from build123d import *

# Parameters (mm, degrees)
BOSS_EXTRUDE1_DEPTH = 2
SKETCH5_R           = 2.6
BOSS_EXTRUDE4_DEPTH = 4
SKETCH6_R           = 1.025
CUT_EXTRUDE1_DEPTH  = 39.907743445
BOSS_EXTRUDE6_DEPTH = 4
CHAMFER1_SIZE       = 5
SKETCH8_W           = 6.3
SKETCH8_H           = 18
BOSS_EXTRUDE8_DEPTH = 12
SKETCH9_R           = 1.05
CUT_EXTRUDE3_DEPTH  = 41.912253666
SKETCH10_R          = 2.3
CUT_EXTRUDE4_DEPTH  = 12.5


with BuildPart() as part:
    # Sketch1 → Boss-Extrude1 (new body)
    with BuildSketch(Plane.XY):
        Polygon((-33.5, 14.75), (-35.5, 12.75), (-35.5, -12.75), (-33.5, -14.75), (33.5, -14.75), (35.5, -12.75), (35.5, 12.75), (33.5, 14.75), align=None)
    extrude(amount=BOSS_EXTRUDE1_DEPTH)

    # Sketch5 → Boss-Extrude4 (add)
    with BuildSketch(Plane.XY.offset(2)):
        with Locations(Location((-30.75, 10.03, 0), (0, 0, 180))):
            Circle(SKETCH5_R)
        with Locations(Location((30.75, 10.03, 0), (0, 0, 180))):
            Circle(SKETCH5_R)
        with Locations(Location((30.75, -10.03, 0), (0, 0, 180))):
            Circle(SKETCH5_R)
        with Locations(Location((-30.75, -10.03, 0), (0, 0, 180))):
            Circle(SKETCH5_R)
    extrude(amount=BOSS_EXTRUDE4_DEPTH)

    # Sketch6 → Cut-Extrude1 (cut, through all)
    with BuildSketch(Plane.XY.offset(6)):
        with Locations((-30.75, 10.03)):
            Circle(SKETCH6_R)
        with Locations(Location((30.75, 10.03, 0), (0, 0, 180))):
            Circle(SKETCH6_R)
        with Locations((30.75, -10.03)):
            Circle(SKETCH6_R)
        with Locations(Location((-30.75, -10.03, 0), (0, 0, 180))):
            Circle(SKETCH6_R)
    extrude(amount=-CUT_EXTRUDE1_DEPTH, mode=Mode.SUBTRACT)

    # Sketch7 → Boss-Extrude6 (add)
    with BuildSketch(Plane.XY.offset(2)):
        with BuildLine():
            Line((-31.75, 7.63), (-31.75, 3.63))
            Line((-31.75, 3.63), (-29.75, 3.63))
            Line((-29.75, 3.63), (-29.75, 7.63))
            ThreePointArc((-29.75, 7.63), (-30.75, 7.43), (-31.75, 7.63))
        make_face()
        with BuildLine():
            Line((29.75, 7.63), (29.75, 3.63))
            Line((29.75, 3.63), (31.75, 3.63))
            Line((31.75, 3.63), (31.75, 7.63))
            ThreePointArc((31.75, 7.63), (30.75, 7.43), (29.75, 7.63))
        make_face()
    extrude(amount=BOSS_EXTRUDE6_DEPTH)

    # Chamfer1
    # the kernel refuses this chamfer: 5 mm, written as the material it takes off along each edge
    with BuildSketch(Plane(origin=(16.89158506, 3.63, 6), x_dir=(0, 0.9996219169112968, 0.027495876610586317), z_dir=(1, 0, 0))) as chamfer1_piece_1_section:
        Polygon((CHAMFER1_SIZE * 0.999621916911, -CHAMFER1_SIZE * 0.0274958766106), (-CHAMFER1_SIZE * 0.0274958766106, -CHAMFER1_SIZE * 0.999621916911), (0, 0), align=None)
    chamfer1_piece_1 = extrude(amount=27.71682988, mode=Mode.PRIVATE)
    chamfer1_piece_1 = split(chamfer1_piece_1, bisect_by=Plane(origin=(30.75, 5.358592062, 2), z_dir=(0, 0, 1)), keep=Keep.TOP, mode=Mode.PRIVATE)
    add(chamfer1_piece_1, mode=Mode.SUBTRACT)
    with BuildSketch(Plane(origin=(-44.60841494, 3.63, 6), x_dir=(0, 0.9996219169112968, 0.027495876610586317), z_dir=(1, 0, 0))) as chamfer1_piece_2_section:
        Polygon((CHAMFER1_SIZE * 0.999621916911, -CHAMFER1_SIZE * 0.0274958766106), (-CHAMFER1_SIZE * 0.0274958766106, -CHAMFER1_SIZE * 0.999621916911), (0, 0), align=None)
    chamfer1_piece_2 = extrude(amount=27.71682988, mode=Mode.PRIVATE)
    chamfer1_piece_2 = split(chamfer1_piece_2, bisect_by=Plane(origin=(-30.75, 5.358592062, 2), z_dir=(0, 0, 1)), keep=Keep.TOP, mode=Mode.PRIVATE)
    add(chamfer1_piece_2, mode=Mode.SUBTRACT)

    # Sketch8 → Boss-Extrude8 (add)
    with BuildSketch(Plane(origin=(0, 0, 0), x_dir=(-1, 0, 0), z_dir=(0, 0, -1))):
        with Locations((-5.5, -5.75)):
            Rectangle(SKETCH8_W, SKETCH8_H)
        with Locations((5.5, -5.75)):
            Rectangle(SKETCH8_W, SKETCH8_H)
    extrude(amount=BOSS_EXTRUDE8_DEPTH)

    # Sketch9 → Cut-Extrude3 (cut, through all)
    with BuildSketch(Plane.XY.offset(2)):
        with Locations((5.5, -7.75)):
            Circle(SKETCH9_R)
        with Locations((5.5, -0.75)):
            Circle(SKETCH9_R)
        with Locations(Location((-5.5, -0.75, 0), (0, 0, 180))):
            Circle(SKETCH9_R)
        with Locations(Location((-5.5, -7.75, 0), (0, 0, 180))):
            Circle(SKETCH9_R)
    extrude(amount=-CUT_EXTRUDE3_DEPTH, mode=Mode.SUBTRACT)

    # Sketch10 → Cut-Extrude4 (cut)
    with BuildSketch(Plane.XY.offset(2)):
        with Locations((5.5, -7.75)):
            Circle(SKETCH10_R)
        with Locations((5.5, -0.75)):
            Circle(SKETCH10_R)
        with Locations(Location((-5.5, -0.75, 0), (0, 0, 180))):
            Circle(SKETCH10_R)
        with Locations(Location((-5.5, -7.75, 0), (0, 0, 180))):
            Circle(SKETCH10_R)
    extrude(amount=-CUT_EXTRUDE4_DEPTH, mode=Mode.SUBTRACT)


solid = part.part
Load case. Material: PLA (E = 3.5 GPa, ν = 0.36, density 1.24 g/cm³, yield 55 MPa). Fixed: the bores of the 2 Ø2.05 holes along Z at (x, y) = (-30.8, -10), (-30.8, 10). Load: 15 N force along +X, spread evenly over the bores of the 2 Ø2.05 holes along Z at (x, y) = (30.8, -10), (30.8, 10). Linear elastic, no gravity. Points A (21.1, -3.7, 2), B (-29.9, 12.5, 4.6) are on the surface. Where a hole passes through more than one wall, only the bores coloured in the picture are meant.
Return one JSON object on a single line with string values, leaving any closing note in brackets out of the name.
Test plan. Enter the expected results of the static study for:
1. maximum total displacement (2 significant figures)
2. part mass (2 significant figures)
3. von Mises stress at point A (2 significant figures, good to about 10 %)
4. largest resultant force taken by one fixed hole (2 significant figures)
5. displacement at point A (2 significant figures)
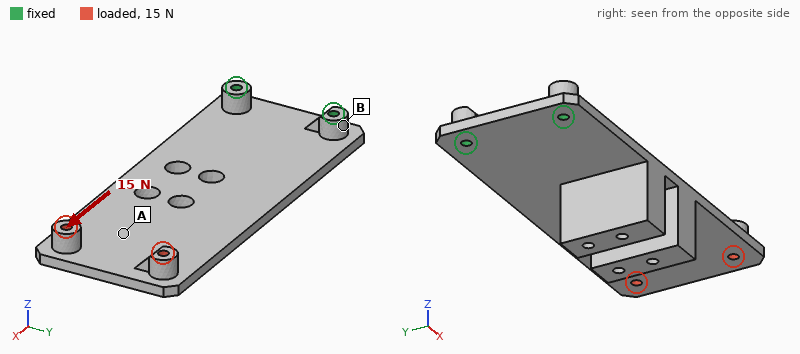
{"maximum total displacement": "0.84 mm", "part mass": "7.8 g", "von Mises stress at point A": "1.6 MPa", "largest resultant force taken by one fixed hole": "7.7 N", "displacement at point A": "0.52 mm"}
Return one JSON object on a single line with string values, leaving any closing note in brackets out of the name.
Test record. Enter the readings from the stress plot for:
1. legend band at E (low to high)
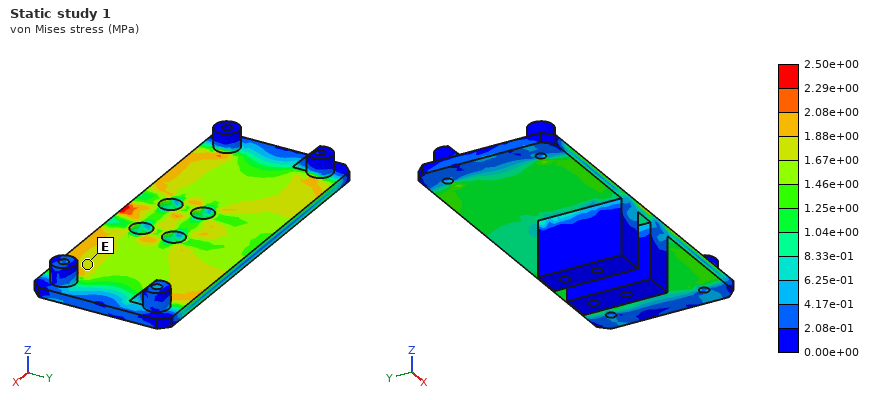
{"legend band at E": "1.67e+00 to 1.88e+00 MPa"}
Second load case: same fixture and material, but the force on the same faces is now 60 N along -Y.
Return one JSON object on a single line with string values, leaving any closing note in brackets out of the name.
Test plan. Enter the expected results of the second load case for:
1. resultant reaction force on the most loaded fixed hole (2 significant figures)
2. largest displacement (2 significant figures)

{"resultant reaction force on the most loaded fixed hole": "180 N", "largest displacement": "0.95 mm"}
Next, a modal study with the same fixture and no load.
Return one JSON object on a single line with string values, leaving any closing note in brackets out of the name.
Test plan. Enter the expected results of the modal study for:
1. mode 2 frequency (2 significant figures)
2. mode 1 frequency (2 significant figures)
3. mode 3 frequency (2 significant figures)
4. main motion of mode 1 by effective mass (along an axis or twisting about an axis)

{"mode 2 frequency": "520 Hz", "mode 1 frequency": "110 Hz", "mode 3 frequency": "670 Hz", "main motion of mode 1 by effective mass": "along Z"}
